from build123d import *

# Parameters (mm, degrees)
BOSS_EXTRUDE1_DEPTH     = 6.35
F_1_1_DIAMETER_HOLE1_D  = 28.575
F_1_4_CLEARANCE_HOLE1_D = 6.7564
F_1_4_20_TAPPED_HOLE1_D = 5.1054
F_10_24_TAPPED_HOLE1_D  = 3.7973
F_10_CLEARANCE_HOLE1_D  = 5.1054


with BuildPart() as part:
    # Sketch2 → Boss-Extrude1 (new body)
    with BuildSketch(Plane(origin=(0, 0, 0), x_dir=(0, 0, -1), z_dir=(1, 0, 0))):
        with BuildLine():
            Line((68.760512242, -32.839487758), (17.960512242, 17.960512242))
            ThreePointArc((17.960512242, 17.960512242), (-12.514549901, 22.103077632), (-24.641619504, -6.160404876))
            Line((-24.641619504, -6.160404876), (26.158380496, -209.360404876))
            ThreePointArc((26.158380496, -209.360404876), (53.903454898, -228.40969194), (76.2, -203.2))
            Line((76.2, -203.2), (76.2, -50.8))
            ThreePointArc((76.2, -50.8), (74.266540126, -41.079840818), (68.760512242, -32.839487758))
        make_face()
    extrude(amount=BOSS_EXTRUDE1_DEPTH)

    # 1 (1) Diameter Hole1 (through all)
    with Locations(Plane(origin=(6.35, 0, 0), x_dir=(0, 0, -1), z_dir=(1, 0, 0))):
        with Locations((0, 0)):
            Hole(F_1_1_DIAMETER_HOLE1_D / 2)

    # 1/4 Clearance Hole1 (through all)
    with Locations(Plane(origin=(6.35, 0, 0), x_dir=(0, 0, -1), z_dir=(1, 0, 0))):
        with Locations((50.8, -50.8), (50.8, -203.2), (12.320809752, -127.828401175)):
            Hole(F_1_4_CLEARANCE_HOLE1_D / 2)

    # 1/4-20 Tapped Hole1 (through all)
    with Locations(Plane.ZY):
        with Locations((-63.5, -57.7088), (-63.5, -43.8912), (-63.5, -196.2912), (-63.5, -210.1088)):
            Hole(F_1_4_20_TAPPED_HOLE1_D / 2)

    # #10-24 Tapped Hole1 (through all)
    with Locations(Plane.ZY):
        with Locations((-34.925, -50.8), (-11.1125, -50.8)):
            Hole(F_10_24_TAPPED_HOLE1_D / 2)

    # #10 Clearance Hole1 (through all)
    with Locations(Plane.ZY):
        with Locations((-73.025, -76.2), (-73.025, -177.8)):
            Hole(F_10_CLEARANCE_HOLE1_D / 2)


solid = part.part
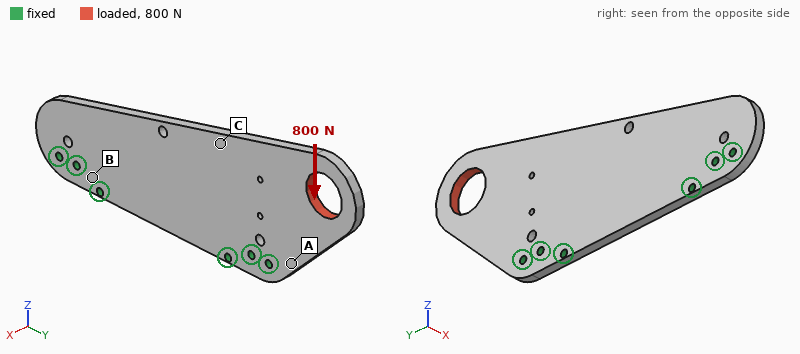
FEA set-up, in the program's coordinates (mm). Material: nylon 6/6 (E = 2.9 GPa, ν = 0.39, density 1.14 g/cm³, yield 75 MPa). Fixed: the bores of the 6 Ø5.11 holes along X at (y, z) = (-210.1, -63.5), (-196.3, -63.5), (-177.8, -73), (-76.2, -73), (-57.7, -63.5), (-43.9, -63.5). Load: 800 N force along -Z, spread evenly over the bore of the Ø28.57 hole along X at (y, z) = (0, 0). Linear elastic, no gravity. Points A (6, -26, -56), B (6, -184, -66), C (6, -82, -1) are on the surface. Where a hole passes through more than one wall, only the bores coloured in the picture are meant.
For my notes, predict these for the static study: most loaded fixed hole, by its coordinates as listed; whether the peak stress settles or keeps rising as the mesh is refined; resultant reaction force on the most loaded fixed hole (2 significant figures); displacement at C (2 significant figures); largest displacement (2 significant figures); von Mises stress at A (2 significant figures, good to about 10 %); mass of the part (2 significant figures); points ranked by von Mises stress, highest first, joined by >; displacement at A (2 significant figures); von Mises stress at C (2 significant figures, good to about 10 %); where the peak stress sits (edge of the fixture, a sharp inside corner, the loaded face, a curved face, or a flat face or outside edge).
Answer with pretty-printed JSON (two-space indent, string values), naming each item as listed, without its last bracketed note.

{
  "most loaded fixed hole, by its coordinates as listed": "(-43.9, -63.5)",
  "whether the peak stress settles or keeps rising as the mesh is refined": "keeps rising",
  "resultant reaction force on the most loaded fixed hole": "960 N",
  "displacement at C": "0.089 mm",
  "largest displacement": "0.52 mm",
  "von Mises stress at A": "6.0 MPa",
  "mass of the part": "120 g",
  "points ranked by von Mises stress, highest first, joined by >": "A > C > B",
  "displacement at A": "0.093 mm",
  "von Mises stress at C": "3.4 MPa",
  "where the peak stress sits": "edge of the fixture"
}
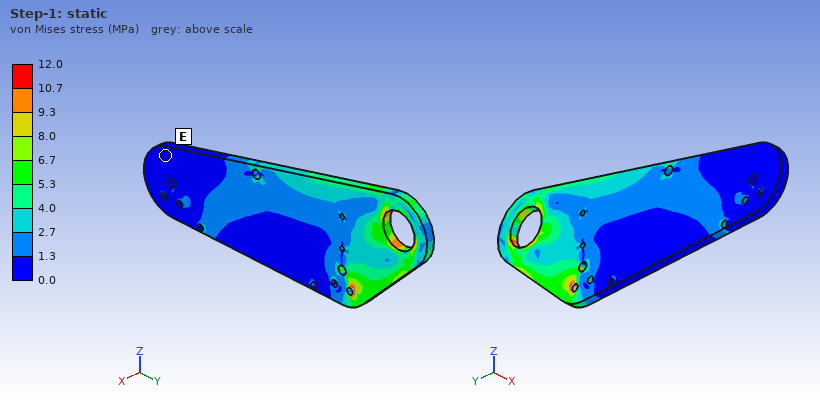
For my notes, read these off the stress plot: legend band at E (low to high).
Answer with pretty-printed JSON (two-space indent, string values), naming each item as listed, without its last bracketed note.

{
  "legend band at E": "0.0 to 1.3 MPa"
}
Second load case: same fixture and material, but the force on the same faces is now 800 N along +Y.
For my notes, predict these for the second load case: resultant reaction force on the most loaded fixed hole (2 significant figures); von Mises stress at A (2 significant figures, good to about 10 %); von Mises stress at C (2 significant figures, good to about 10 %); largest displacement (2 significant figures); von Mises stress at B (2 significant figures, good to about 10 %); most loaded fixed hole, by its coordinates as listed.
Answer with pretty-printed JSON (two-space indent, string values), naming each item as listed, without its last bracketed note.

{
  "resultant reaction force on the most loaded fixed hole": "460 N",
  "von Mises stress at A": "1.5 MPa",
  "von Mises stress at C": "3.7 MPa",
  "largest displacement": "0.40 mm",
  "von Mises stress at B": "1.1 MPa",
  "most loaded fixed hole, by its coordinates as listed": "(-43.9, -63.5)"
}
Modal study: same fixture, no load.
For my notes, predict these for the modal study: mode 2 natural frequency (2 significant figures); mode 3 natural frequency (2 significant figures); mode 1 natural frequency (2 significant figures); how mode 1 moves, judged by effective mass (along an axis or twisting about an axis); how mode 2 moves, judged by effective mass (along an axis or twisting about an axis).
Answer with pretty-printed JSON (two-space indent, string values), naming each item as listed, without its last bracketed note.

{
  "mode 2 natural frequency": "330 Hz",
  "mode 3 natural frequency": "600 Hz",
  "mode 1 natural frequency": "200 Hz",
  "how mode 1 moves, judged by effective mass": "along X",
  "how mode 2 moves, judged by effective mass": "along X"
}
